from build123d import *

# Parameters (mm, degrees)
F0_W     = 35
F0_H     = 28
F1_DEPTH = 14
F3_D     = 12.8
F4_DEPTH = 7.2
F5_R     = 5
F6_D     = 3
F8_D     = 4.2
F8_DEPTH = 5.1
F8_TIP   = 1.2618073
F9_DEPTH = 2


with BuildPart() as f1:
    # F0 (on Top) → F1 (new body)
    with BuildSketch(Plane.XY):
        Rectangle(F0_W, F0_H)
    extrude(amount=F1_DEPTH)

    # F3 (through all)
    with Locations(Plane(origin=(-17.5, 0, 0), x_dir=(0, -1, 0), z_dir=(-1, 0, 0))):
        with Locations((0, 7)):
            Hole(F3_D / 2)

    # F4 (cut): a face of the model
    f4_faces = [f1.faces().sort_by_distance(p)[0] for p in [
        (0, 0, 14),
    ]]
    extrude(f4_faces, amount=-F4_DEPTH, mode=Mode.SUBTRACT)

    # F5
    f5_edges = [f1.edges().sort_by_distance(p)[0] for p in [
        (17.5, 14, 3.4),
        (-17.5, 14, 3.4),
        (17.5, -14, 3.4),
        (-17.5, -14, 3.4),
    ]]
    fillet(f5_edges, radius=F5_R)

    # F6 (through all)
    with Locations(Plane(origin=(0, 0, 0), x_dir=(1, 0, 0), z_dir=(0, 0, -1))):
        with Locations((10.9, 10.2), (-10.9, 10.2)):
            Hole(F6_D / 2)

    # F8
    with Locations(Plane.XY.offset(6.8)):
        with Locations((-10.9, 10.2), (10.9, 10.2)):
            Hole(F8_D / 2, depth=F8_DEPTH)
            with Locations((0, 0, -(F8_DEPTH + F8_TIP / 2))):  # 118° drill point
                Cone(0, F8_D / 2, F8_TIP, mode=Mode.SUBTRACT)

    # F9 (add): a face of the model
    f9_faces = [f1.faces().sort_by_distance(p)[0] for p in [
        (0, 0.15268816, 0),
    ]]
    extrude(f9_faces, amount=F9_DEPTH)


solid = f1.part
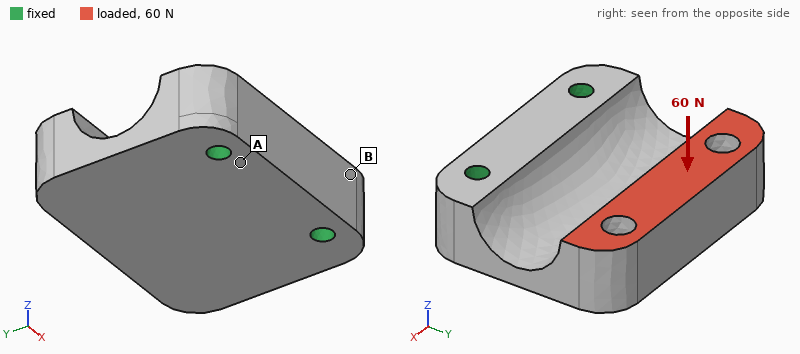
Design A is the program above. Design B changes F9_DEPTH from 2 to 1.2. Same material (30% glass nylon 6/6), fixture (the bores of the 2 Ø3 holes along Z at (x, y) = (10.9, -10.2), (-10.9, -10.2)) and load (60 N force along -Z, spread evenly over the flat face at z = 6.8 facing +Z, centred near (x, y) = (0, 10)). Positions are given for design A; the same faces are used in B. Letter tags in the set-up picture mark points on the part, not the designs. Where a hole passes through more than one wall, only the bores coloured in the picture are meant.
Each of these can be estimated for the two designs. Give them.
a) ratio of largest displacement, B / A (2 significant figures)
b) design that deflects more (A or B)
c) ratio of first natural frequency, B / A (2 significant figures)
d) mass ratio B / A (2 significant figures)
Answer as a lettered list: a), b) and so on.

a) 2.3
b) B
c) 0.70
d) 0.87
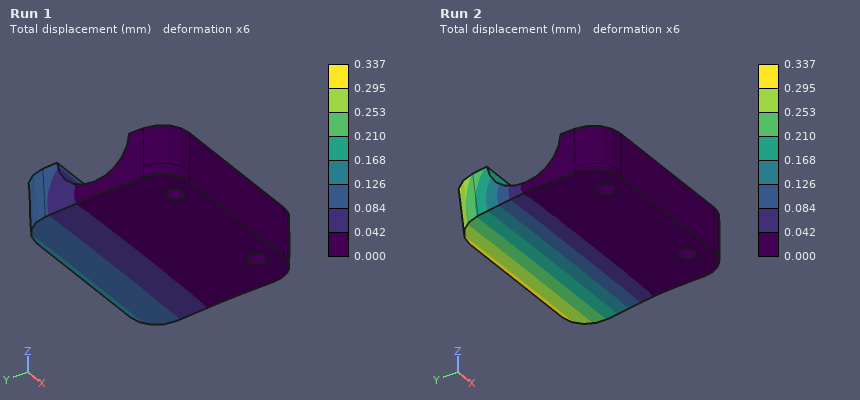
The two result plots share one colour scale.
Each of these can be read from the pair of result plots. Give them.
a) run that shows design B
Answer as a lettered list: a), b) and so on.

a) Run 2
